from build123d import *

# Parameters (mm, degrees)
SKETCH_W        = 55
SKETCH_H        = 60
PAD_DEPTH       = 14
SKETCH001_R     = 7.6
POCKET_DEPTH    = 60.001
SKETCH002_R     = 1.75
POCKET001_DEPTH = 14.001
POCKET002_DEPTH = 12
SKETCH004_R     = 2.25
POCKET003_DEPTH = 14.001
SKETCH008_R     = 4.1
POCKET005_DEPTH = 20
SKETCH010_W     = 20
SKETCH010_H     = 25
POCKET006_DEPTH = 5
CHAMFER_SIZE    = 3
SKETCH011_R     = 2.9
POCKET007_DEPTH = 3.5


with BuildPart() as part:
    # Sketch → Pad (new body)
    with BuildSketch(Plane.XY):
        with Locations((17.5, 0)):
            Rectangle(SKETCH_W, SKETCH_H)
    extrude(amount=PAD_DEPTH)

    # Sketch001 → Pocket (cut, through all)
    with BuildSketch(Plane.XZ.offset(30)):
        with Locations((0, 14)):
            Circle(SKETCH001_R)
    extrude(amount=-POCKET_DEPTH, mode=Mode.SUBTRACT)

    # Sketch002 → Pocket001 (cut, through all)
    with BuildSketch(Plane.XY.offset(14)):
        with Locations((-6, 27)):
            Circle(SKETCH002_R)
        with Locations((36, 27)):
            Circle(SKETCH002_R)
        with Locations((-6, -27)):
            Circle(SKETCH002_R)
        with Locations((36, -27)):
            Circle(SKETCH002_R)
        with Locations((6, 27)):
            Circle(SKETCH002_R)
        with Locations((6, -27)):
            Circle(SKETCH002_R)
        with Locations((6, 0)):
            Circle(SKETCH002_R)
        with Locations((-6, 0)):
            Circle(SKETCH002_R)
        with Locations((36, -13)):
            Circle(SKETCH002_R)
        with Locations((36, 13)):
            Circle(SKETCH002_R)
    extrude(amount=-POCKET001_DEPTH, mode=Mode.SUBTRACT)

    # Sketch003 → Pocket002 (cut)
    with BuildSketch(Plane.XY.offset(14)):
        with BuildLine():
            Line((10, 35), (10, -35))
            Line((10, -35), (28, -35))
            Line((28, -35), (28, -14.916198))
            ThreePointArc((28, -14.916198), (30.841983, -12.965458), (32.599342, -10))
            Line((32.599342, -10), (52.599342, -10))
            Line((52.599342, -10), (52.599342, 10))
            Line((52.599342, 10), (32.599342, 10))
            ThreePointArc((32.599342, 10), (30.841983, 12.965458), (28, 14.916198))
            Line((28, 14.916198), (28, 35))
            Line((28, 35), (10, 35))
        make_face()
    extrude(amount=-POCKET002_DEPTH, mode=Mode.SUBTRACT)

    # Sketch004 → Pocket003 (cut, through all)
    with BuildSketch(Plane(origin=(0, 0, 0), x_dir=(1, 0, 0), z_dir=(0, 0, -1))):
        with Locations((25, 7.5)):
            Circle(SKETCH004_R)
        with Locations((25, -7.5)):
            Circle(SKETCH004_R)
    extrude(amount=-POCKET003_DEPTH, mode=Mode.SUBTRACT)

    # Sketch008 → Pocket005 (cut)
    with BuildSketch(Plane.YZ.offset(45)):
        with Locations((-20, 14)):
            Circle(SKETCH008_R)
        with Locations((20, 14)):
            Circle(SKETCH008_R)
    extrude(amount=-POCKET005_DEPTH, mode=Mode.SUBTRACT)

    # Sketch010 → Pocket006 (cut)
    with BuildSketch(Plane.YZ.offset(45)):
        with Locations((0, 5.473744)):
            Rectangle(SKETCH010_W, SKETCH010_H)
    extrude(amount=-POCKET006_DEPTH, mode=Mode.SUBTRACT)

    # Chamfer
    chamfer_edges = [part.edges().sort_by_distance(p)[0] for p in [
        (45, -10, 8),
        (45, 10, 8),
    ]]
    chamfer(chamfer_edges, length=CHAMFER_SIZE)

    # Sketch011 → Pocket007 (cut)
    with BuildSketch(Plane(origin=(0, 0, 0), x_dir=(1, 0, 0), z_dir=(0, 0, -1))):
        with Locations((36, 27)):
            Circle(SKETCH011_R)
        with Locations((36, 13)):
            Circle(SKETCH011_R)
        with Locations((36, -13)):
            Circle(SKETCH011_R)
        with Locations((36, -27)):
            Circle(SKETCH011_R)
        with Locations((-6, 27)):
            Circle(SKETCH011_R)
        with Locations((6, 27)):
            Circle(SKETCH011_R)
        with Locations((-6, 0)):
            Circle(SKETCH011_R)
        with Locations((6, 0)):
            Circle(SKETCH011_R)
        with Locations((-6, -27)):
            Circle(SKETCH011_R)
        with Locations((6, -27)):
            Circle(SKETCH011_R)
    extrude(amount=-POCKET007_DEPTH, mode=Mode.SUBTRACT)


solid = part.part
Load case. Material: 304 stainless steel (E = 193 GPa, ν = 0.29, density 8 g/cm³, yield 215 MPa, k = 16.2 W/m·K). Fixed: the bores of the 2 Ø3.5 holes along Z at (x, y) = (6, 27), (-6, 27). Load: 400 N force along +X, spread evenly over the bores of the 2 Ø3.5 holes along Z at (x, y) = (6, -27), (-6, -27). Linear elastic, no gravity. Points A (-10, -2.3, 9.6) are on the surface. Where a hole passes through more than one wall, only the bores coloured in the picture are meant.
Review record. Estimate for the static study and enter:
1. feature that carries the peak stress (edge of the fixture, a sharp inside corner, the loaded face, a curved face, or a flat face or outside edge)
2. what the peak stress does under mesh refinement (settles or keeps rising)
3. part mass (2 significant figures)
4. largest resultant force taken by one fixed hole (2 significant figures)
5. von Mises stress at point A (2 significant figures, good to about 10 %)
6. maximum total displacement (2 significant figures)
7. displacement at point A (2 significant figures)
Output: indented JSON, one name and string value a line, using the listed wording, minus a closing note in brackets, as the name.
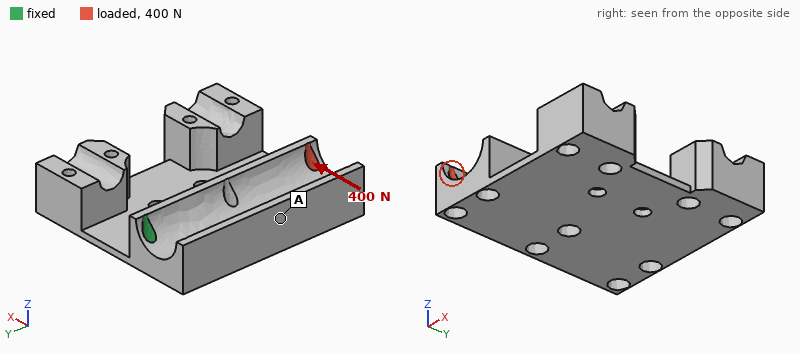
{
  "feature that carries the peak stress": "edge of the fixture",
  "what the peak stress does under mesh refinement": "keeps rising",
  "part mass": "160 g",
  "largest resultant force taken by one fixed hole": "1.4 kN",
  "von Mises stress at point A": "10 MPa",
  "maximum total displacement": "32 µm",
  "displacement at point A": "11 µm"
}
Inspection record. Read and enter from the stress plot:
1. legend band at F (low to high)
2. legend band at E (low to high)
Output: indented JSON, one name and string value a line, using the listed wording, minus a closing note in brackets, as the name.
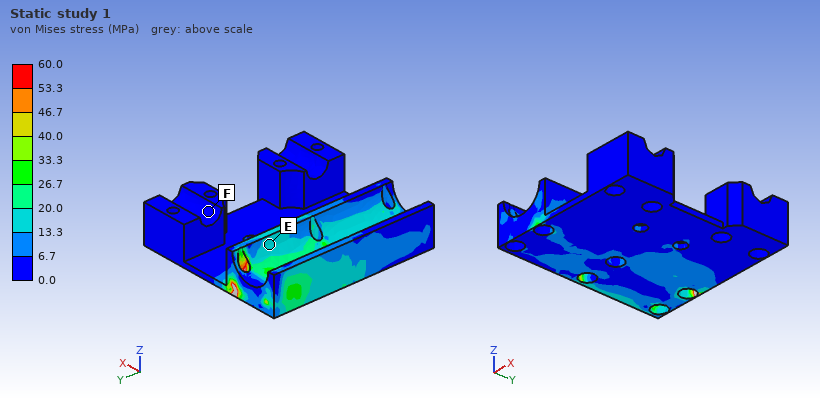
{
  "legend band at F": "0.0 to 6.7 MPa",
  "legend band at E": "13.3 to 20.0 MPa"
}
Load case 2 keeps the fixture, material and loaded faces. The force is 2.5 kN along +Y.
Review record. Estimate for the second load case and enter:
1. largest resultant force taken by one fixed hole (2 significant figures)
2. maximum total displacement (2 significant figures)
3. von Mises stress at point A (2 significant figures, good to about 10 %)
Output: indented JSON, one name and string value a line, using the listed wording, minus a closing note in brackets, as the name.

{
  "largest resultant force taken by one fixed hole": "1.3 kN",
  "maximum total displacement": "18 µm",
  "von Mises stress at point A": "29 MPa"
}
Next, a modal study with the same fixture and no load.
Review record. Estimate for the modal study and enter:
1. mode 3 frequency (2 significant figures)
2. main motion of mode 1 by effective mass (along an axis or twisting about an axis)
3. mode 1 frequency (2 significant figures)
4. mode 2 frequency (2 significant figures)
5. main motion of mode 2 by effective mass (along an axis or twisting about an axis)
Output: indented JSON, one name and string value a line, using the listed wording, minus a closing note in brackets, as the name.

{
  "mode 3 frequency": "2200 Hz",
  "main motion of mode 1 by effective mass": "along Z",
  "mode 1 frequency": "580 Hz",
  "mode 2 frequency": "940 Hz",
  "main motion of mode 2 by effective mass": "twisting about X"
}
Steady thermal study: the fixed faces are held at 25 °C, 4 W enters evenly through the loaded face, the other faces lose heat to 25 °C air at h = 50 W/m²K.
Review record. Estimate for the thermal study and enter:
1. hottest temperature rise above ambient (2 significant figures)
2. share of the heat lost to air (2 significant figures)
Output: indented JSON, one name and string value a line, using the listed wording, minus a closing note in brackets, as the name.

{
  "hottest temperature rise above ambient": "32 K",
  "share of the heat lost to air": "85 %"
}
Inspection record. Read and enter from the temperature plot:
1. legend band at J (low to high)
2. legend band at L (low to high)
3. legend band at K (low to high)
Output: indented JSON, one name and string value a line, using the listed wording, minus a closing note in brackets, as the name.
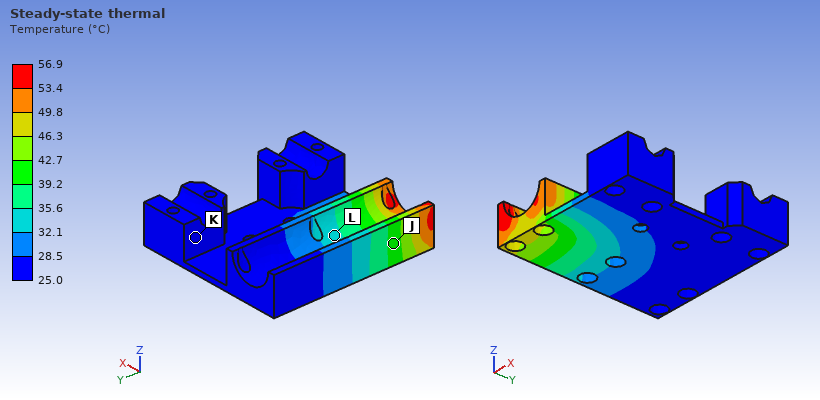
{
  "legend band at J": "39.2 to 42.7 °C",
  "legend band at L": "32.1 to 35.6 °C",
  "legend band at K": "25.0 to 28.5 °C"
}
